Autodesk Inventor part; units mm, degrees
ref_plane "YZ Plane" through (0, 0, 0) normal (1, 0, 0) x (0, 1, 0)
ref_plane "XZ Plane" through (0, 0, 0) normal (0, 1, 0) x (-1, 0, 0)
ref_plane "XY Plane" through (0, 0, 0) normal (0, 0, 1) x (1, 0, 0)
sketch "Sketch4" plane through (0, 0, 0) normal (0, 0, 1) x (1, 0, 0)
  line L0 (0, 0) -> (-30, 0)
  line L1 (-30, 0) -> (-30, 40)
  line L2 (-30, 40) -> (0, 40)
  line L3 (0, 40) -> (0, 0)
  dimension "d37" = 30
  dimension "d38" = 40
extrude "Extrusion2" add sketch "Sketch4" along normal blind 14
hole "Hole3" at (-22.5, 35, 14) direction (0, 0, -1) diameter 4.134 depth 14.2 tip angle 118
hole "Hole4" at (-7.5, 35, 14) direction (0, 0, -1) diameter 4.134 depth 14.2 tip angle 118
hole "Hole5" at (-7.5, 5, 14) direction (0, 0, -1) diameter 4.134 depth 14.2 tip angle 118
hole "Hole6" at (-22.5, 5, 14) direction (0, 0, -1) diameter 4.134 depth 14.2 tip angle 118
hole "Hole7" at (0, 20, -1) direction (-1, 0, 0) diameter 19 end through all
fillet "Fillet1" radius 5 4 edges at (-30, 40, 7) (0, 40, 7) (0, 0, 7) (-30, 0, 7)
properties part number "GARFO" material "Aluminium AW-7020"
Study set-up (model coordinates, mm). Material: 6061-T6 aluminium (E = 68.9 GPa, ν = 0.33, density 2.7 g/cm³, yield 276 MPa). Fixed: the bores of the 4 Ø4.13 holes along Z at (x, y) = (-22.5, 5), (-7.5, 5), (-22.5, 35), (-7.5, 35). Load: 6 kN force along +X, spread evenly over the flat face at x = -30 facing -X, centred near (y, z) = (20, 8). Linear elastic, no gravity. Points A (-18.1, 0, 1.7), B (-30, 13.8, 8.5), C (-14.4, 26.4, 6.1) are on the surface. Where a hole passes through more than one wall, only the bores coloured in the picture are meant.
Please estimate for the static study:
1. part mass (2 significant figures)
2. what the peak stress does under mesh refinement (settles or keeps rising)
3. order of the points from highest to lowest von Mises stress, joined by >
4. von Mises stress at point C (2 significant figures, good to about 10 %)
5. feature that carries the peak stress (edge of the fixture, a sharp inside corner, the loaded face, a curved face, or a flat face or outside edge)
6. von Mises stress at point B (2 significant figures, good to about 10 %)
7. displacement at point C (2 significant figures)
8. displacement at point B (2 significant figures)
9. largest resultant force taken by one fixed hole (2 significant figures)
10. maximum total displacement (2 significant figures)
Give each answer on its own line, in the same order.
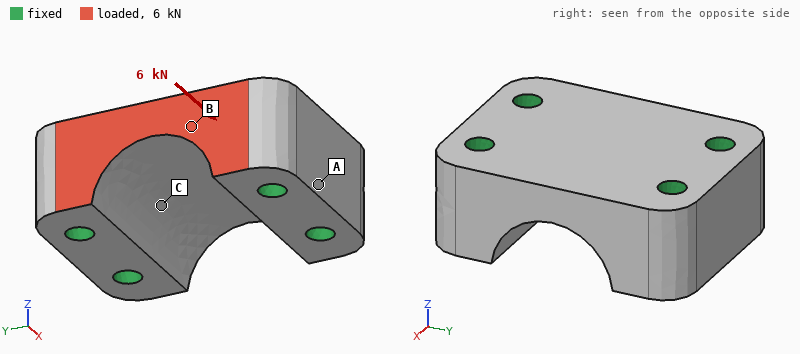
33 g
keeps rising
B > C > A
11 MPa
edge of the fixture
20 MPa
1.4 µm
5.1 µm
2.2 kN
7.0 µm
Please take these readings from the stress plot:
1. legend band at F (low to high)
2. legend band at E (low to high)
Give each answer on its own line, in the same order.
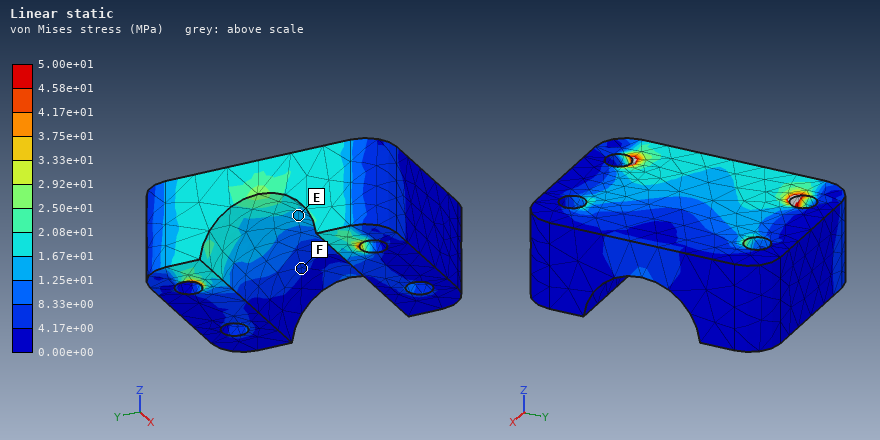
4.17e+00 to 8.33e+00 MPa
1.25e+01 to 1.67e+01 MPa
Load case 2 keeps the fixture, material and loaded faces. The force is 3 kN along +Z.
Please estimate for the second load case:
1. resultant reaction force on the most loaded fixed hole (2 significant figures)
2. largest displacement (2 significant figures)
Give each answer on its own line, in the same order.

1.6 kN
12 µm
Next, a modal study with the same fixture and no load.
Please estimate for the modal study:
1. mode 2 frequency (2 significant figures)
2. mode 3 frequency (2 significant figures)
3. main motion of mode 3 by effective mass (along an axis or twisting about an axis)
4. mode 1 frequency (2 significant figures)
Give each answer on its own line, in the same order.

48 kHz
58 kHz
along X
48 kHz
